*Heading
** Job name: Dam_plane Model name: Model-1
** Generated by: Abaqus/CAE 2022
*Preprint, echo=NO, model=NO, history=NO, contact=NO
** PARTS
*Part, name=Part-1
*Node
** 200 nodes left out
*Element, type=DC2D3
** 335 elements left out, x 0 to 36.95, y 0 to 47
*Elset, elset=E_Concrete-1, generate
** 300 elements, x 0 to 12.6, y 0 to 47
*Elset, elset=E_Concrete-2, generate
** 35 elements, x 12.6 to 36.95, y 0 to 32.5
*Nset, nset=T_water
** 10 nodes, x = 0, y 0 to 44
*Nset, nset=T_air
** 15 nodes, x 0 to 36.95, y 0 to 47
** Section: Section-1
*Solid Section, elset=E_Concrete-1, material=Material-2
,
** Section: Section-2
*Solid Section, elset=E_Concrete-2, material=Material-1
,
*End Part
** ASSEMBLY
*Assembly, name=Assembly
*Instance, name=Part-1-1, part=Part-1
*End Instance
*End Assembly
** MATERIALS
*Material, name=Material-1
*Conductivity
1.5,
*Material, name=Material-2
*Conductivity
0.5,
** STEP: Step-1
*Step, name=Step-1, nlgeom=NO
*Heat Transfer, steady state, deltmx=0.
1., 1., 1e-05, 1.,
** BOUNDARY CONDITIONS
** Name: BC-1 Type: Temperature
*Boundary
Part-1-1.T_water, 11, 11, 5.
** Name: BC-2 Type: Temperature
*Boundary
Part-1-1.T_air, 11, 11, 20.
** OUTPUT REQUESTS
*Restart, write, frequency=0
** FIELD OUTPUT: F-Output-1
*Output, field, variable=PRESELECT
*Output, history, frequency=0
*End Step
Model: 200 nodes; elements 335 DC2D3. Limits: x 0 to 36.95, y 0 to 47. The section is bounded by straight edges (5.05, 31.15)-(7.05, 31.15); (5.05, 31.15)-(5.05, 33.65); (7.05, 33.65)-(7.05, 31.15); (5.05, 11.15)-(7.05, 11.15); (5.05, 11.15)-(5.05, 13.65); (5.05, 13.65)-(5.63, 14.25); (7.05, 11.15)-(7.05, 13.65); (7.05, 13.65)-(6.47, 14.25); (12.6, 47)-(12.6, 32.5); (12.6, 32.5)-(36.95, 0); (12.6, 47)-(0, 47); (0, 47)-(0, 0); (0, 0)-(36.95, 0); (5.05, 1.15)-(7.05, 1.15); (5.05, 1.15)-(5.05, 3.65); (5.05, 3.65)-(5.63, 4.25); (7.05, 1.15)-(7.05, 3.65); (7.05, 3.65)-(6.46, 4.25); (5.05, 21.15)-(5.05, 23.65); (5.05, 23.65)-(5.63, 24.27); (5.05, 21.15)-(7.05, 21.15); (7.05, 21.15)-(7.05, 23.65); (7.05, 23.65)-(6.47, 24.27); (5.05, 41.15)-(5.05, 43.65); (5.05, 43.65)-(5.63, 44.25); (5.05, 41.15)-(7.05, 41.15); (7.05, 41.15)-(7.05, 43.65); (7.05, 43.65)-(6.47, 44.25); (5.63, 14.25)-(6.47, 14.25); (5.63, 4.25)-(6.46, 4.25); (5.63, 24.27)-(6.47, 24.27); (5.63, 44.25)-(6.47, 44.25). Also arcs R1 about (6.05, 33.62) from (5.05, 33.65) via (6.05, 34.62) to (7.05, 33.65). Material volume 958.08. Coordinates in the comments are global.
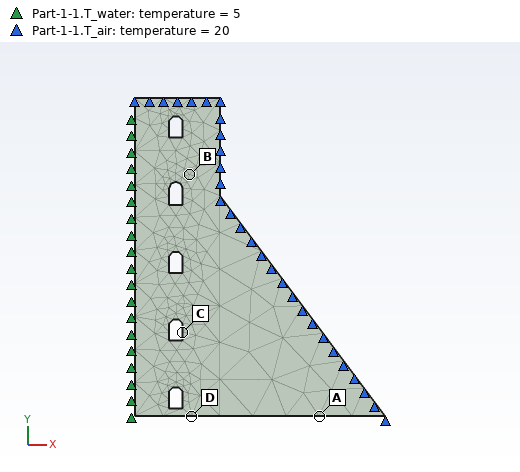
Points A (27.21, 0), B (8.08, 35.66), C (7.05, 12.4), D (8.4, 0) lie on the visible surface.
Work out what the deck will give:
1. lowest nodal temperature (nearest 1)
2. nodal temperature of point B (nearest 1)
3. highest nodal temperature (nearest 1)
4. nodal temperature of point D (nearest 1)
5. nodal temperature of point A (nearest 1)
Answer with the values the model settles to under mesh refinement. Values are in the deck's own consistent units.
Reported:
5
15
20
13
19
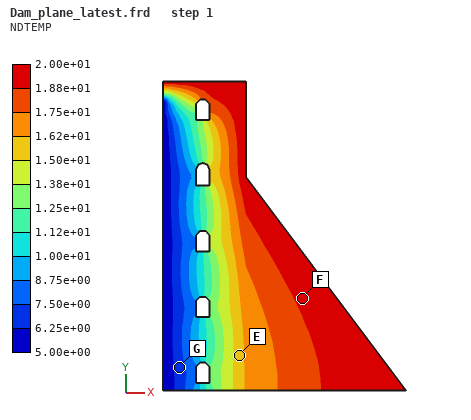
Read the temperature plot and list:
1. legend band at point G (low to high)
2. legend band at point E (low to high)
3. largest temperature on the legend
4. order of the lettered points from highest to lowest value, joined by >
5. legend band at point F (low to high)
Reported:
6.25e+00 to 7.50e+00
1.50e+01 to 1.62e+01
2.00e+01
F > E > G
1.88e+01 to 2.00e+01
